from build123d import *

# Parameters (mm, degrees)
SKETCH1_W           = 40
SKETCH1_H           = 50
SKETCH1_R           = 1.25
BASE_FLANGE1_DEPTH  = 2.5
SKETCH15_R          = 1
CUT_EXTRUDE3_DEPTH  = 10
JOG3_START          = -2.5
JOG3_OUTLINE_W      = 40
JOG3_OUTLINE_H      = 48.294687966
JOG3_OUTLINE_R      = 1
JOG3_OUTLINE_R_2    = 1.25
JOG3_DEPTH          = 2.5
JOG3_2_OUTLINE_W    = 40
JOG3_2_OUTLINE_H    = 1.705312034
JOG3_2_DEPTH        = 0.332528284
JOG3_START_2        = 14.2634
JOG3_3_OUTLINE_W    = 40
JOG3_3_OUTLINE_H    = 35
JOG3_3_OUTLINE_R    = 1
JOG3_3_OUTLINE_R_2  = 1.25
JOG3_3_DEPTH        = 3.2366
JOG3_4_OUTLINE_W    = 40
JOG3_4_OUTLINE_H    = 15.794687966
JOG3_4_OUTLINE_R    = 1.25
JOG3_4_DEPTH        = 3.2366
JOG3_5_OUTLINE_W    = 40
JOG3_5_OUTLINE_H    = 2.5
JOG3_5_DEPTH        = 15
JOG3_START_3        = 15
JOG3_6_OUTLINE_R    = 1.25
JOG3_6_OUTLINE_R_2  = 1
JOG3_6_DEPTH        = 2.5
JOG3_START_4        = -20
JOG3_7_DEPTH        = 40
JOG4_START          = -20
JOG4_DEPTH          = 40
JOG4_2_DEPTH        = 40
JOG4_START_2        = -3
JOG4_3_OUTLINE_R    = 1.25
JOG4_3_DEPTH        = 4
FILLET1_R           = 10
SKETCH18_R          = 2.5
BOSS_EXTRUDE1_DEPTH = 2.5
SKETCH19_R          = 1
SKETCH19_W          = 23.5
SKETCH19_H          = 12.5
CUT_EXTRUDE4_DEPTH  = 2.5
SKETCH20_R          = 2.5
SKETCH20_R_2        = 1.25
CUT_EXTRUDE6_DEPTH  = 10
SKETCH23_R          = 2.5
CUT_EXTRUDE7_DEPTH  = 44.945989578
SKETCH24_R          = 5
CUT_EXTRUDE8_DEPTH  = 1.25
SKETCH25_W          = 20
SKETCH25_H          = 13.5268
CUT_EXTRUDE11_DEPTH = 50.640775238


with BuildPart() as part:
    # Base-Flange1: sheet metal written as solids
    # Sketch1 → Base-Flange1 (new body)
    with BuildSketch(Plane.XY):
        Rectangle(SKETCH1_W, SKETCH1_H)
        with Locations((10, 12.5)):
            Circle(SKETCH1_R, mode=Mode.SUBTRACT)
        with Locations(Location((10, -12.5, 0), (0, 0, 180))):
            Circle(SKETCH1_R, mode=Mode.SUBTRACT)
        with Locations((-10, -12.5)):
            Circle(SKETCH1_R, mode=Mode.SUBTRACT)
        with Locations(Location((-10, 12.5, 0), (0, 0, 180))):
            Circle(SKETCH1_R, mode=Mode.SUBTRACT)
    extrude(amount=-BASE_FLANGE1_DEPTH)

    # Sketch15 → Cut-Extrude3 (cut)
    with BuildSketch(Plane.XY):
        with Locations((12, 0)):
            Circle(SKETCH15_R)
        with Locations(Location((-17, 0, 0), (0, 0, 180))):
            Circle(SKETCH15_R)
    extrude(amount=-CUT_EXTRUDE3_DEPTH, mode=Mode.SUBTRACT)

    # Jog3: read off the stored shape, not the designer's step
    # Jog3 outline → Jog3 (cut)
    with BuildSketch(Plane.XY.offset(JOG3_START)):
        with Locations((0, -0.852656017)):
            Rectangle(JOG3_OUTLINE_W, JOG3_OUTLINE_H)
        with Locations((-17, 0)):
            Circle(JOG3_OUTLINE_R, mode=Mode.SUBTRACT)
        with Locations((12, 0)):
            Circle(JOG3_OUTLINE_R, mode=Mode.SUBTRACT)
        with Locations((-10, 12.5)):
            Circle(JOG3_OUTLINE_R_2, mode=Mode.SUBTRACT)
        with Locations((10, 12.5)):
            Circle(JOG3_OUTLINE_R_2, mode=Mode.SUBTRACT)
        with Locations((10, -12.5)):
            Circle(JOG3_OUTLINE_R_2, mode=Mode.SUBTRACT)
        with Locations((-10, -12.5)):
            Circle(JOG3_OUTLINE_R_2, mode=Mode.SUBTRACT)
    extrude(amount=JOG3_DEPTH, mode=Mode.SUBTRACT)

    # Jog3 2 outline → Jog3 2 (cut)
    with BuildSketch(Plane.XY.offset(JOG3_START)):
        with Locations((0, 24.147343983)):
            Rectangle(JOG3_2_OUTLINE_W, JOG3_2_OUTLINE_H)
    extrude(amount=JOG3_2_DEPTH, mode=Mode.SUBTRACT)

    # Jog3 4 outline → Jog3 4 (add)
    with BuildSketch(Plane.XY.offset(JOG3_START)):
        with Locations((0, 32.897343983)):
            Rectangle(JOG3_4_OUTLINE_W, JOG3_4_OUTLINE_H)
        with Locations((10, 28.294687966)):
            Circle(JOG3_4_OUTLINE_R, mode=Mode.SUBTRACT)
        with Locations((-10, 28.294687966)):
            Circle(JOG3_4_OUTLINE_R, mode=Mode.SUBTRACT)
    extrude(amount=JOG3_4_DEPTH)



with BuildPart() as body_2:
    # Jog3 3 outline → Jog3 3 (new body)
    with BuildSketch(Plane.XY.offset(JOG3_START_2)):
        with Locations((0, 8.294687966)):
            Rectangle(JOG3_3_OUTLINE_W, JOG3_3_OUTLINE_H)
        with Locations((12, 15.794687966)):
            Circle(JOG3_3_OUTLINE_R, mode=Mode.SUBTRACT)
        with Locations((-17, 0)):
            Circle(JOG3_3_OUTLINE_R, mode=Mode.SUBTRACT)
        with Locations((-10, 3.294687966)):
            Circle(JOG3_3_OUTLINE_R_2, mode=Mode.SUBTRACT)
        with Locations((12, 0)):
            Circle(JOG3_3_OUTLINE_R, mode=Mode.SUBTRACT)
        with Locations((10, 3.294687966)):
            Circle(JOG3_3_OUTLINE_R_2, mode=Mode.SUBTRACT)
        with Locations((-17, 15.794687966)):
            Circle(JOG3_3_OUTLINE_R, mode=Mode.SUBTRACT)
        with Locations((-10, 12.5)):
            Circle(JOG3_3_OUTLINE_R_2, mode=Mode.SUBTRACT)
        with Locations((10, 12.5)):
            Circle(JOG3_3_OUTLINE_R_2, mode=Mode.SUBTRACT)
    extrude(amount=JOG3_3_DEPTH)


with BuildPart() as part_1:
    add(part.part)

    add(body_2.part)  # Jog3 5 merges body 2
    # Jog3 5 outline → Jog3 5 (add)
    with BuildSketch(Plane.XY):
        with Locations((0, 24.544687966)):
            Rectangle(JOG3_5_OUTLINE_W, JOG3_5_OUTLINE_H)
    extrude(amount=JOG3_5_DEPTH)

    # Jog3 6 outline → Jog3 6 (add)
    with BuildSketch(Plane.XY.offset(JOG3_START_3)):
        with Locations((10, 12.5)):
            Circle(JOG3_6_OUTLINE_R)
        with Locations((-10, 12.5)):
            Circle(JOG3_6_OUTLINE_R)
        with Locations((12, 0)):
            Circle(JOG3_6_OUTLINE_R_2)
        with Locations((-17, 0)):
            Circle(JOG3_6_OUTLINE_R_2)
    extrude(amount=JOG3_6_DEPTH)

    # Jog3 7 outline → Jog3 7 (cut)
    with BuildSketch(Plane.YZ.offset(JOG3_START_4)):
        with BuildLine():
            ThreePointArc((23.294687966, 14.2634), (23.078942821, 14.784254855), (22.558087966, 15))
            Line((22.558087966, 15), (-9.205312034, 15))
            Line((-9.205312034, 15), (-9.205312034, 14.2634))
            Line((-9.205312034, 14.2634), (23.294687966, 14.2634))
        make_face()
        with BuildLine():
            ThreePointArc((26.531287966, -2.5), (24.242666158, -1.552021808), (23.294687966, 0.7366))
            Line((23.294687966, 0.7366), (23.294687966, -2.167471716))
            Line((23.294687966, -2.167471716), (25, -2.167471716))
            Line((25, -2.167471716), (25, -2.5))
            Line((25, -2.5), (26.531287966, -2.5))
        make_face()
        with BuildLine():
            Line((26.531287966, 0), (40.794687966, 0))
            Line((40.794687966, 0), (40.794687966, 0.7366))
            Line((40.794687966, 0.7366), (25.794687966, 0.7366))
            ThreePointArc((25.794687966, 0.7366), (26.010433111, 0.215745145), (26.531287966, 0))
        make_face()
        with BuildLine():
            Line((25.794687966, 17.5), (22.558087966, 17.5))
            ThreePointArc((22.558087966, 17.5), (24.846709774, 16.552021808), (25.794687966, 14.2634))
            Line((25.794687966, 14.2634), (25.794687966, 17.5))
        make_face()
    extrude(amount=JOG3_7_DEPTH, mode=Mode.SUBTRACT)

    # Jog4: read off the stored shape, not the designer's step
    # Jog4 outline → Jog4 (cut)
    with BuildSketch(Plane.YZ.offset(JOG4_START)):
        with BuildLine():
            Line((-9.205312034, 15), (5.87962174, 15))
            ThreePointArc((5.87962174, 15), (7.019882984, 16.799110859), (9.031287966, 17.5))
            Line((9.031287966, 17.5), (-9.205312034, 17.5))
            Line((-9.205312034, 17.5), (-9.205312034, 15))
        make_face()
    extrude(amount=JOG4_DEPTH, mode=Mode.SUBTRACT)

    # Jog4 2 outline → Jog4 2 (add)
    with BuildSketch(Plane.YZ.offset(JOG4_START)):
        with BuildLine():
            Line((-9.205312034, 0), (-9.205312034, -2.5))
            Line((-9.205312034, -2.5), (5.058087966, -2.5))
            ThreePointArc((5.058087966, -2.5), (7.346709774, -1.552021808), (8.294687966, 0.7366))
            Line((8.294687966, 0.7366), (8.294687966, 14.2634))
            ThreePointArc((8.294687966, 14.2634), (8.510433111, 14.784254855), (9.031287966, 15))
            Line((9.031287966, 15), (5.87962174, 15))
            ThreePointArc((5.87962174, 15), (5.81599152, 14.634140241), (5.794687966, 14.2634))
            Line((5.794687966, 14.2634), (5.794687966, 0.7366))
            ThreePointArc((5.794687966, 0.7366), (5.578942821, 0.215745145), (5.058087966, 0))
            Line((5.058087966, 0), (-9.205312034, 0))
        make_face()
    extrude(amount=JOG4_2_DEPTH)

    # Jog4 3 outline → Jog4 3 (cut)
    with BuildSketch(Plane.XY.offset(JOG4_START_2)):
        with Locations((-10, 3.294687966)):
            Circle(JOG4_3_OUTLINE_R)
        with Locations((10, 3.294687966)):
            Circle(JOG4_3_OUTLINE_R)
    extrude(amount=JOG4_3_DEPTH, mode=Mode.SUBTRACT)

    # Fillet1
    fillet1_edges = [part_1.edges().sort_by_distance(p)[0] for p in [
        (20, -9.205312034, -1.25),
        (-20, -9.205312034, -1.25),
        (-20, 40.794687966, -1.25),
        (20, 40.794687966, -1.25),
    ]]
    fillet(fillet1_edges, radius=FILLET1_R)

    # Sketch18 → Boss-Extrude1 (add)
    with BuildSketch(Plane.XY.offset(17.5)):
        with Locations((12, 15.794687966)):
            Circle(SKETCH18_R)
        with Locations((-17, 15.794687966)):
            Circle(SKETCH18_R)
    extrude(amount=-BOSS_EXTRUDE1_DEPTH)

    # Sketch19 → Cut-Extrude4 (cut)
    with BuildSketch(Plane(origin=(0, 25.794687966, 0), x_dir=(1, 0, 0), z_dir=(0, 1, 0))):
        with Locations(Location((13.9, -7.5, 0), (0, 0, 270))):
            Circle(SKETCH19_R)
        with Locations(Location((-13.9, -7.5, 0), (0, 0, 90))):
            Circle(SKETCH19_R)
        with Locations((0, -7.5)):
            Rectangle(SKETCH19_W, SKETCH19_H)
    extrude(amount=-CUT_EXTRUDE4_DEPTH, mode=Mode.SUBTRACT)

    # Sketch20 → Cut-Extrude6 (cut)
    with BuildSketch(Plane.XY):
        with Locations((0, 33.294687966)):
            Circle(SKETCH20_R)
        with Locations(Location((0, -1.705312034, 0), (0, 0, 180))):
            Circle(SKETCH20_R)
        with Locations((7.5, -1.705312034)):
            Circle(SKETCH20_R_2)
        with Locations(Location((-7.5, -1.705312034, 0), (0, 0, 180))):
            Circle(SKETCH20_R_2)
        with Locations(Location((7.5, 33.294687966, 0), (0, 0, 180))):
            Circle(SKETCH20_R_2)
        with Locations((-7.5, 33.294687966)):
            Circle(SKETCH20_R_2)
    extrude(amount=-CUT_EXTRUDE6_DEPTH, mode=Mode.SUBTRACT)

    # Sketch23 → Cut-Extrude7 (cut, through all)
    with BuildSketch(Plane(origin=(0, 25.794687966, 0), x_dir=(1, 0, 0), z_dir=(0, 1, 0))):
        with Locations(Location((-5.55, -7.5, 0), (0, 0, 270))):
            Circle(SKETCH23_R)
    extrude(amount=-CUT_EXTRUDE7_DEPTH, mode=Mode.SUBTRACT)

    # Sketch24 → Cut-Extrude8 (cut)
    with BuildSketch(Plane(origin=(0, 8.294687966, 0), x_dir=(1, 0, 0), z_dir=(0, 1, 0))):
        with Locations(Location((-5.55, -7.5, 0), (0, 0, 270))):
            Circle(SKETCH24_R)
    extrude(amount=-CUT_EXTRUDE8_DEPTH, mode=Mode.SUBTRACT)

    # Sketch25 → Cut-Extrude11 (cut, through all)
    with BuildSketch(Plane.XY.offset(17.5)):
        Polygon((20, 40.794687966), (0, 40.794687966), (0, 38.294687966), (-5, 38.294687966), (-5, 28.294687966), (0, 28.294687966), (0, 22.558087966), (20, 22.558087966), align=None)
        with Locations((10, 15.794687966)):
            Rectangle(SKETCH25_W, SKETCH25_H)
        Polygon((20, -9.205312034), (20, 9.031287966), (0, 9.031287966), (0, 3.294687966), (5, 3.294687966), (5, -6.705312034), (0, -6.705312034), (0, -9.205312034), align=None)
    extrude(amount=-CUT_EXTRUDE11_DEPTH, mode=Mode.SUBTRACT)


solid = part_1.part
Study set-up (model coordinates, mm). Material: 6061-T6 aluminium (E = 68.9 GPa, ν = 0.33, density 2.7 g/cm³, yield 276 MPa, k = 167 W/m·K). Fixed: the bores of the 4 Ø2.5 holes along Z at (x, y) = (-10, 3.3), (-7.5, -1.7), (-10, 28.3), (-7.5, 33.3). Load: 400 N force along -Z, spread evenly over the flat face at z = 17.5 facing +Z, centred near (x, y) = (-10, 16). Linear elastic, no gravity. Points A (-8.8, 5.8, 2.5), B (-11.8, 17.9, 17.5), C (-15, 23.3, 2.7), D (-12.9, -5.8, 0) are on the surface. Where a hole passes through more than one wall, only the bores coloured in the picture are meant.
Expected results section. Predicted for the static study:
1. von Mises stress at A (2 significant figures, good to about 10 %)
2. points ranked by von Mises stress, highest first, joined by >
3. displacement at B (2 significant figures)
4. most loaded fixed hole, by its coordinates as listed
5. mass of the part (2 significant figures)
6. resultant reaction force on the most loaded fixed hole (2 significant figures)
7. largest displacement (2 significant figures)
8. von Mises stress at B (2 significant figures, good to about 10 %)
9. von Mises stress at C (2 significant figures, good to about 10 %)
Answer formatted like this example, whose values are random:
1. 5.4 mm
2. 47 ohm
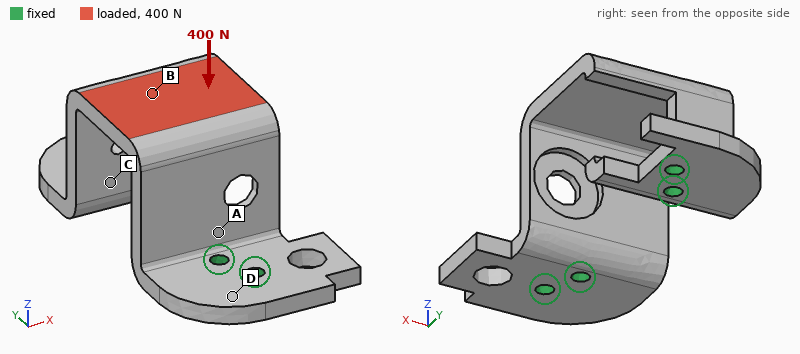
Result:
1. 20 MPa
2. B > A > C > D
3. 26 µm
4. (-10, 28.3)
5. 9.1 g
6. 220 N
7. 57 µm
8. 30 MPa
9. 12 MPa
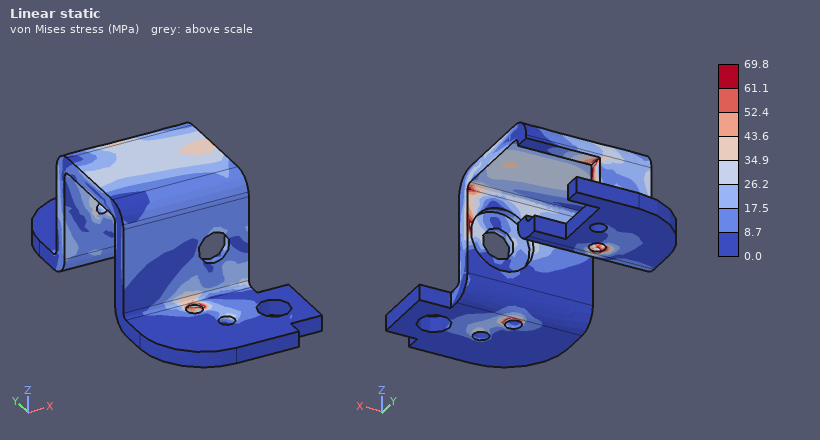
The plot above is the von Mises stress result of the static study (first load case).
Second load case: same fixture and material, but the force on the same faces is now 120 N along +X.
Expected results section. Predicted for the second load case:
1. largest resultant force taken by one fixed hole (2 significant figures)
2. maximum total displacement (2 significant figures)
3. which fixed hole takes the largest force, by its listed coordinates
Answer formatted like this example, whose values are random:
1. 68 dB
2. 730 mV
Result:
1. 140 N
2. 62 µm
3. (-10, 3.3)
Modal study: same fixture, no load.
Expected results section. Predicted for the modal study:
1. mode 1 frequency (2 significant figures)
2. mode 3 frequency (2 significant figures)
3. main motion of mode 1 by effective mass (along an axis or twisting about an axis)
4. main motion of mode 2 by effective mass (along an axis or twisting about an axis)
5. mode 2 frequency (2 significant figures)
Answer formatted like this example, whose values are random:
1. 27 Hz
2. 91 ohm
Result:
1. 4300 Hz
2. 7300 Hz
3. along X
4. along Y
5. 4700 Hz
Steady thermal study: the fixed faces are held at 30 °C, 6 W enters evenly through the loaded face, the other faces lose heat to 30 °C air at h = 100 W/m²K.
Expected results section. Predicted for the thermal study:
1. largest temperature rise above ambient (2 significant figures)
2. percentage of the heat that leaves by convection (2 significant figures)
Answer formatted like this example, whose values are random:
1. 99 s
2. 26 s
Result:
1. 13 K
2. 24 %
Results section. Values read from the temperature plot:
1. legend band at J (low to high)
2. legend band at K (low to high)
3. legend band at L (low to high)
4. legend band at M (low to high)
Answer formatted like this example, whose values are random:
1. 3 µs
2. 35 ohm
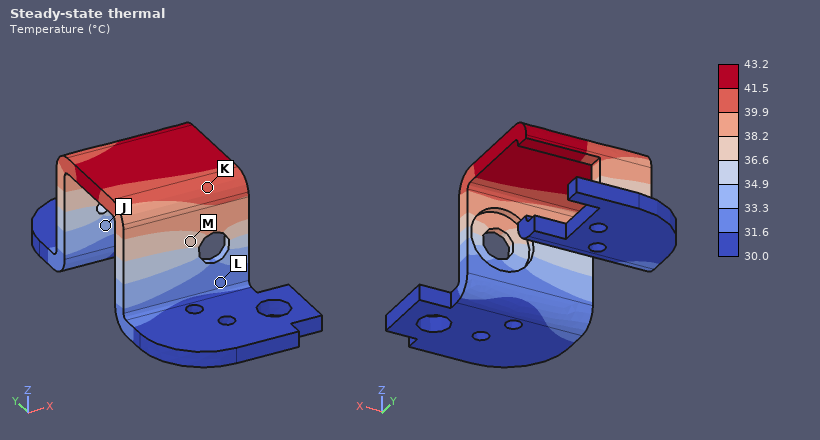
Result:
1. 33.3 to 34.9 °C
2. 39.9 to 41.5 °C
3. 31.6 to 33.3 °C
4. 36.6 to 38.2 °C
